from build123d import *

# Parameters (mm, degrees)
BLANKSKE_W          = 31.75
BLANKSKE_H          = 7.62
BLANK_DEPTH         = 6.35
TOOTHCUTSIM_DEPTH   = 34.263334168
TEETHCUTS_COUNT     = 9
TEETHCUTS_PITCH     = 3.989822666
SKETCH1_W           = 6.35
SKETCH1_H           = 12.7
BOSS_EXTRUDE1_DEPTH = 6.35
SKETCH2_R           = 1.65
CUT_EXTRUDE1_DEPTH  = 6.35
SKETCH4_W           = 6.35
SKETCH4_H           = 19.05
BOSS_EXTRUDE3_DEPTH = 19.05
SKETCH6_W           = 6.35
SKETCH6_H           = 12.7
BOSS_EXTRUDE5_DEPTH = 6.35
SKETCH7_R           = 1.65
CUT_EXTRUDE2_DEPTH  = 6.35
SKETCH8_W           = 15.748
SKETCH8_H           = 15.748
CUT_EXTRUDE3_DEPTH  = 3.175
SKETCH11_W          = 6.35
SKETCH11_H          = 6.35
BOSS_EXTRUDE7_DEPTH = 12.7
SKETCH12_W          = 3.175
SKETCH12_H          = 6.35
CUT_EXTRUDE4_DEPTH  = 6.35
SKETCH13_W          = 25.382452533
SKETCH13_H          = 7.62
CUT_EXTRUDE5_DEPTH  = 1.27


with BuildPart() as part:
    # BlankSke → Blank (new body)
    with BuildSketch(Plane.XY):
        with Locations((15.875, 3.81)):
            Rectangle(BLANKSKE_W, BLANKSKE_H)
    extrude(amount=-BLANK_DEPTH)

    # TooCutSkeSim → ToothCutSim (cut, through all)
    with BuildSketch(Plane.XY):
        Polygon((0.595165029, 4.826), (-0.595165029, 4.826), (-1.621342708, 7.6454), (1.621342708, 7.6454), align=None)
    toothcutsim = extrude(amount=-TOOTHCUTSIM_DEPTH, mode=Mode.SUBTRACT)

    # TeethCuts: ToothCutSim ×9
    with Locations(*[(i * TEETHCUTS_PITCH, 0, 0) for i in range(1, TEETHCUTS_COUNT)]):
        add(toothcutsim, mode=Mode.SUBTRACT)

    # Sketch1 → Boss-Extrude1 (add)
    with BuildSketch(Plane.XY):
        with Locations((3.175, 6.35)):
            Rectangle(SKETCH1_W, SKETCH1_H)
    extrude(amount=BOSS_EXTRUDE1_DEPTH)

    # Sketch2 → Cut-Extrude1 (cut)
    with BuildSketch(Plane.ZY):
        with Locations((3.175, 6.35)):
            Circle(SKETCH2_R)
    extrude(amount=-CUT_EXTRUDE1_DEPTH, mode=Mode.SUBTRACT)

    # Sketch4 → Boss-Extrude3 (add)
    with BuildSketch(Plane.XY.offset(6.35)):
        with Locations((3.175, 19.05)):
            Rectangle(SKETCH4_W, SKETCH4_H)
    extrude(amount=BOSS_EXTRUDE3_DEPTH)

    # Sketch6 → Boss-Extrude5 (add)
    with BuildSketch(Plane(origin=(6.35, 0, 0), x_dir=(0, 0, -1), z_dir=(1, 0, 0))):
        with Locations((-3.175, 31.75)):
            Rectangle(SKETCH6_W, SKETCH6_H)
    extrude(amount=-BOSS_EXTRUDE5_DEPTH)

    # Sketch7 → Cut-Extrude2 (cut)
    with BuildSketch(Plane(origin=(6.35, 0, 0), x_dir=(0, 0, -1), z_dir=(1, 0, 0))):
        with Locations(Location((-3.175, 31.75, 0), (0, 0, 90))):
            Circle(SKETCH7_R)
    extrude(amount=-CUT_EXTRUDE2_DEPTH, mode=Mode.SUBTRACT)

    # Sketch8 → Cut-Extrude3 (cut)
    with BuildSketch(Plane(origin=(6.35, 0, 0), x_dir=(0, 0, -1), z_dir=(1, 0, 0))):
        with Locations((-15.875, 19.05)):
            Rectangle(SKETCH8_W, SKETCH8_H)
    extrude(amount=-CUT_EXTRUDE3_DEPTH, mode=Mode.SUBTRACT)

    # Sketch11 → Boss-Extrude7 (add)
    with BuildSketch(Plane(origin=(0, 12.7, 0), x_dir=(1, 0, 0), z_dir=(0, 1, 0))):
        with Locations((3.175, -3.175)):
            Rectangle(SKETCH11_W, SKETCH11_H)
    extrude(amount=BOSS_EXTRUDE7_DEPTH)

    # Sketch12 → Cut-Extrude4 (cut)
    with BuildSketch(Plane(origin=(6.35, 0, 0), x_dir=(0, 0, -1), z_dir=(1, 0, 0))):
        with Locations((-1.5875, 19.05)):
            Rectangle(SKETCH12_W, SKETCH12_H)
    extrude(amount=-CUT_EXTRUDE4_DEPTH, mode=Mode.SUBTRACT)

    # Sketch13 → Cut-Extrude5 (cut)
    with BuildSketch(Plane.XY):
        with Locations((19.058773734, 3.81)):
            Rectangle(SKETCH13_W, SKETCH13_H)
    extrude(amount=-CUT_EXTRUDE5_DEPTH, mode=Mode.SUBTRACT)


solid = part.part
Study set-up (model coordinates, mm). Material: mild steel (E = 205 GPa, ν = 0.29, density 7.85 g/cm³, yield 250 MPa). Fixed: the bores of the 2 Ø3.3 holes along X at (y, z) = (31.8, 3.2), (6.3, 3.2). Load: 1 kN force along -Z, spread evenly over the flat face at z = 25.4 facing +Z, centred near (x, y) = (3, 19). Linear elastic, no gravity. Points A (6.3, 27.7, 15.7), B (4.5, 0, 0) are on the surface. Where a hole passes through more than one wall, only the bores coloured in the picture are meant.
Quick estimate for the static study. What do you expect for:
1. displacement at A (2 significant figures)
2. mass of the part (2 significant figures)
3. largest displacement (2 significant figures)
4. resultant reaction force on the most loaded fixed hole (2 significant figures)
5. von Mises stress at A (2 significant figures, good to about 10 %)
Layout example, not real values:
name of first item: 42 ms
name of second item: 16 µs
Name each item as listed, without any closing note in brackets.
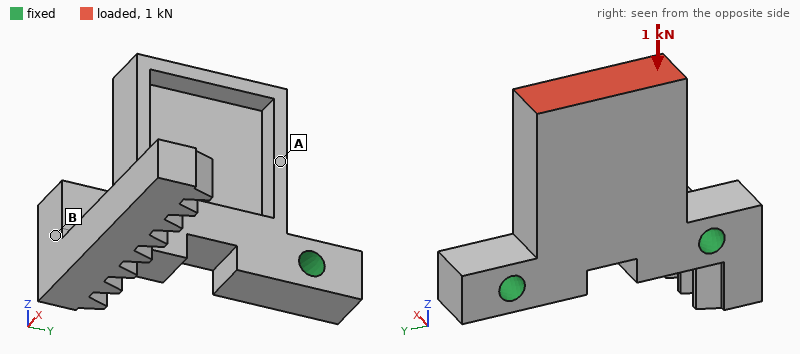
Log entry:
displacement at A: 3.2 µm
mass of the part: 30 g
largest displacement: 11 µm
resultant reaction force on the most loaded fixed hole: 560 N
von Mises stress at A: 45 MPa
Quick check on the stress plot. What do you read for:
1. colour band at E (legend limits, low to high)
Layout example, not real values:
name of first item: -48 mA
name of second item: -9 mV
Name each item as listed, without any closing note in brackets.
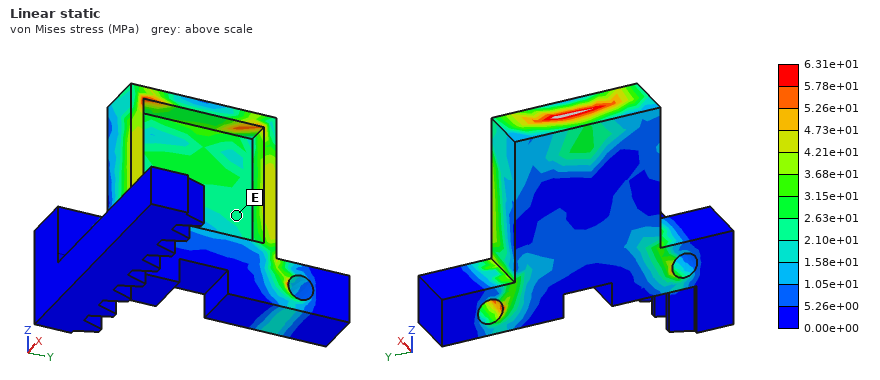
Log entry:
colour band at E: 2.10e+01 to 2.63e+01 MPa
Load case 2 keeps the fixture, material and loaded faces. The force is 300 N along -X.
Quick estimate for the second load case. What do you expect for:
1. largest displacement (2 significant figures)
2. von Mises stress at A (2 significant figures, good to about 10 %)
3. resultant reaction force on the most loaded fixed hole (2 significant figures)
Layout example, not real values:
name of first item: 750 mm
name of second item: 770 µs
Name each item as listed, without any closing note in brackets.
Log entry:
largest displacement: 46 µm
von Mises stress at A: 82 MPa
resultant reaction force on the most loaded fixed hole: 180 N
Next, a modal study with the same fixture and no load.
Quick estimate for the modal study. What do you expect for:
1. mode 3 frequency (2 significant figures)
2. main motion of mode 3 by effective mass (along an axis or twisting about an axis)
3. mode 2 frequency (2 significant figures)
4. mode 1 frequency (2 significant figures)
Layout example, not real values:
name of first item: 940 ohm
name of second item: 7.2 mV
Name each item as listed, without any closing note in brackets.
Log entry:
mode 3 frequency: 6700 Hz
main motion of mode 3 by effective mass: along X
mode 2 frequency: 4200 Hz
mode 1 frequency: 3900 Hz
